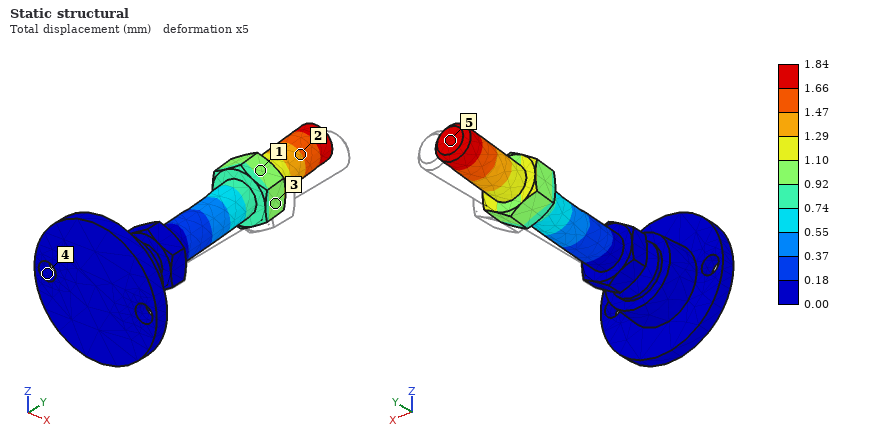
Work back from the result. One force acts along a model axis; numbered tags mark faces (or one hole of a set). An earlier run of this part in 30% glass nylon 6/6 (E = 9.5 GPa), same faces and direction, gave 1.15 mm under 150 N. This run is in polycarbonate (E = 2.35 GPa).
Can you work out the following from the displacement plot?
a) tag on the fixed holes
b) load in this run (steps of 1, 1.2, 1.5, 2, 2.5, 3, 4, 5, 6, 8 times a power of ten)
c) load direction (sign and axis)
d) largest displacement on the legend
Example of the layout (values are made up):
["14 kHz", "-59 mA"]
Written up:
["4", "60 N", "-X", "1.84 mm"]
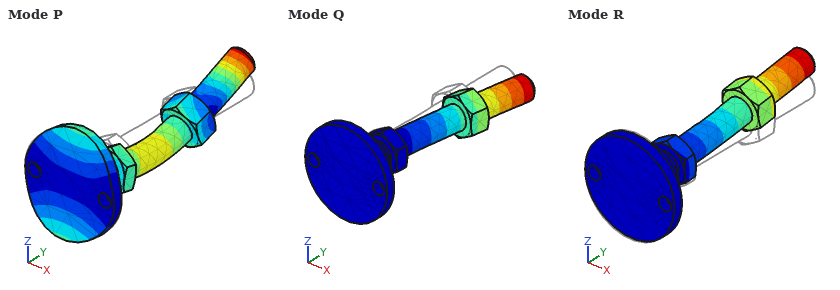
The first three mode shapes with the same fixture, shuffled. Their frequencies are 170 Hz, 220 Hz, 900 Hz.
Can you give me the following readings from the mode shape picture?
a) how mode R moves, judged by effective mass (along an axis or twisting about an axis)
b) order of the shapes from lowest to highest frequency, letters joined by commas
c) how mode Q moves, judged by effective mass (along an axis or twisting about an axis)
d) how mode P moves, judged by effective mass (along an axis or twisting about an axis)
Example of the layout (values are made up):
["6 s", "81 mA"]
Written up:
["along Z", "R, Q, P", "along X", "along Z"]
